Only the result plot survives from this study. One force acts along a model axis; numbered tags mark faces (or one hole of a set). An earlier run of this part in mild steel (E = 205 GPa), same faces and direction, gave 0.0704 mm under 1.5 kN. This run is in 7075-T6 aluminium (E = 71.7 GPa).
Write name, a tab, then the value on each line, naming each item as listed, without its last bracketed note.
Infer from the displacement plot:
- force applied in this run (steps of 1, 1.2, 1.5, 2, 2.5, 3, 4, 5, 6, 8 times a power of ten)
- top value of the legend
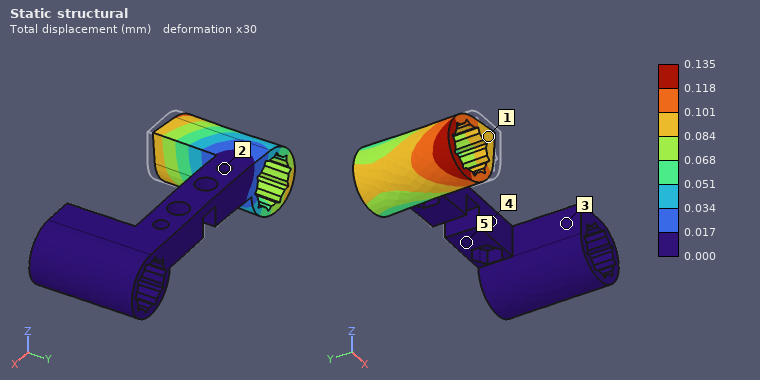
force applied in this run	1 kN
top value of the legend	0.135 mm
